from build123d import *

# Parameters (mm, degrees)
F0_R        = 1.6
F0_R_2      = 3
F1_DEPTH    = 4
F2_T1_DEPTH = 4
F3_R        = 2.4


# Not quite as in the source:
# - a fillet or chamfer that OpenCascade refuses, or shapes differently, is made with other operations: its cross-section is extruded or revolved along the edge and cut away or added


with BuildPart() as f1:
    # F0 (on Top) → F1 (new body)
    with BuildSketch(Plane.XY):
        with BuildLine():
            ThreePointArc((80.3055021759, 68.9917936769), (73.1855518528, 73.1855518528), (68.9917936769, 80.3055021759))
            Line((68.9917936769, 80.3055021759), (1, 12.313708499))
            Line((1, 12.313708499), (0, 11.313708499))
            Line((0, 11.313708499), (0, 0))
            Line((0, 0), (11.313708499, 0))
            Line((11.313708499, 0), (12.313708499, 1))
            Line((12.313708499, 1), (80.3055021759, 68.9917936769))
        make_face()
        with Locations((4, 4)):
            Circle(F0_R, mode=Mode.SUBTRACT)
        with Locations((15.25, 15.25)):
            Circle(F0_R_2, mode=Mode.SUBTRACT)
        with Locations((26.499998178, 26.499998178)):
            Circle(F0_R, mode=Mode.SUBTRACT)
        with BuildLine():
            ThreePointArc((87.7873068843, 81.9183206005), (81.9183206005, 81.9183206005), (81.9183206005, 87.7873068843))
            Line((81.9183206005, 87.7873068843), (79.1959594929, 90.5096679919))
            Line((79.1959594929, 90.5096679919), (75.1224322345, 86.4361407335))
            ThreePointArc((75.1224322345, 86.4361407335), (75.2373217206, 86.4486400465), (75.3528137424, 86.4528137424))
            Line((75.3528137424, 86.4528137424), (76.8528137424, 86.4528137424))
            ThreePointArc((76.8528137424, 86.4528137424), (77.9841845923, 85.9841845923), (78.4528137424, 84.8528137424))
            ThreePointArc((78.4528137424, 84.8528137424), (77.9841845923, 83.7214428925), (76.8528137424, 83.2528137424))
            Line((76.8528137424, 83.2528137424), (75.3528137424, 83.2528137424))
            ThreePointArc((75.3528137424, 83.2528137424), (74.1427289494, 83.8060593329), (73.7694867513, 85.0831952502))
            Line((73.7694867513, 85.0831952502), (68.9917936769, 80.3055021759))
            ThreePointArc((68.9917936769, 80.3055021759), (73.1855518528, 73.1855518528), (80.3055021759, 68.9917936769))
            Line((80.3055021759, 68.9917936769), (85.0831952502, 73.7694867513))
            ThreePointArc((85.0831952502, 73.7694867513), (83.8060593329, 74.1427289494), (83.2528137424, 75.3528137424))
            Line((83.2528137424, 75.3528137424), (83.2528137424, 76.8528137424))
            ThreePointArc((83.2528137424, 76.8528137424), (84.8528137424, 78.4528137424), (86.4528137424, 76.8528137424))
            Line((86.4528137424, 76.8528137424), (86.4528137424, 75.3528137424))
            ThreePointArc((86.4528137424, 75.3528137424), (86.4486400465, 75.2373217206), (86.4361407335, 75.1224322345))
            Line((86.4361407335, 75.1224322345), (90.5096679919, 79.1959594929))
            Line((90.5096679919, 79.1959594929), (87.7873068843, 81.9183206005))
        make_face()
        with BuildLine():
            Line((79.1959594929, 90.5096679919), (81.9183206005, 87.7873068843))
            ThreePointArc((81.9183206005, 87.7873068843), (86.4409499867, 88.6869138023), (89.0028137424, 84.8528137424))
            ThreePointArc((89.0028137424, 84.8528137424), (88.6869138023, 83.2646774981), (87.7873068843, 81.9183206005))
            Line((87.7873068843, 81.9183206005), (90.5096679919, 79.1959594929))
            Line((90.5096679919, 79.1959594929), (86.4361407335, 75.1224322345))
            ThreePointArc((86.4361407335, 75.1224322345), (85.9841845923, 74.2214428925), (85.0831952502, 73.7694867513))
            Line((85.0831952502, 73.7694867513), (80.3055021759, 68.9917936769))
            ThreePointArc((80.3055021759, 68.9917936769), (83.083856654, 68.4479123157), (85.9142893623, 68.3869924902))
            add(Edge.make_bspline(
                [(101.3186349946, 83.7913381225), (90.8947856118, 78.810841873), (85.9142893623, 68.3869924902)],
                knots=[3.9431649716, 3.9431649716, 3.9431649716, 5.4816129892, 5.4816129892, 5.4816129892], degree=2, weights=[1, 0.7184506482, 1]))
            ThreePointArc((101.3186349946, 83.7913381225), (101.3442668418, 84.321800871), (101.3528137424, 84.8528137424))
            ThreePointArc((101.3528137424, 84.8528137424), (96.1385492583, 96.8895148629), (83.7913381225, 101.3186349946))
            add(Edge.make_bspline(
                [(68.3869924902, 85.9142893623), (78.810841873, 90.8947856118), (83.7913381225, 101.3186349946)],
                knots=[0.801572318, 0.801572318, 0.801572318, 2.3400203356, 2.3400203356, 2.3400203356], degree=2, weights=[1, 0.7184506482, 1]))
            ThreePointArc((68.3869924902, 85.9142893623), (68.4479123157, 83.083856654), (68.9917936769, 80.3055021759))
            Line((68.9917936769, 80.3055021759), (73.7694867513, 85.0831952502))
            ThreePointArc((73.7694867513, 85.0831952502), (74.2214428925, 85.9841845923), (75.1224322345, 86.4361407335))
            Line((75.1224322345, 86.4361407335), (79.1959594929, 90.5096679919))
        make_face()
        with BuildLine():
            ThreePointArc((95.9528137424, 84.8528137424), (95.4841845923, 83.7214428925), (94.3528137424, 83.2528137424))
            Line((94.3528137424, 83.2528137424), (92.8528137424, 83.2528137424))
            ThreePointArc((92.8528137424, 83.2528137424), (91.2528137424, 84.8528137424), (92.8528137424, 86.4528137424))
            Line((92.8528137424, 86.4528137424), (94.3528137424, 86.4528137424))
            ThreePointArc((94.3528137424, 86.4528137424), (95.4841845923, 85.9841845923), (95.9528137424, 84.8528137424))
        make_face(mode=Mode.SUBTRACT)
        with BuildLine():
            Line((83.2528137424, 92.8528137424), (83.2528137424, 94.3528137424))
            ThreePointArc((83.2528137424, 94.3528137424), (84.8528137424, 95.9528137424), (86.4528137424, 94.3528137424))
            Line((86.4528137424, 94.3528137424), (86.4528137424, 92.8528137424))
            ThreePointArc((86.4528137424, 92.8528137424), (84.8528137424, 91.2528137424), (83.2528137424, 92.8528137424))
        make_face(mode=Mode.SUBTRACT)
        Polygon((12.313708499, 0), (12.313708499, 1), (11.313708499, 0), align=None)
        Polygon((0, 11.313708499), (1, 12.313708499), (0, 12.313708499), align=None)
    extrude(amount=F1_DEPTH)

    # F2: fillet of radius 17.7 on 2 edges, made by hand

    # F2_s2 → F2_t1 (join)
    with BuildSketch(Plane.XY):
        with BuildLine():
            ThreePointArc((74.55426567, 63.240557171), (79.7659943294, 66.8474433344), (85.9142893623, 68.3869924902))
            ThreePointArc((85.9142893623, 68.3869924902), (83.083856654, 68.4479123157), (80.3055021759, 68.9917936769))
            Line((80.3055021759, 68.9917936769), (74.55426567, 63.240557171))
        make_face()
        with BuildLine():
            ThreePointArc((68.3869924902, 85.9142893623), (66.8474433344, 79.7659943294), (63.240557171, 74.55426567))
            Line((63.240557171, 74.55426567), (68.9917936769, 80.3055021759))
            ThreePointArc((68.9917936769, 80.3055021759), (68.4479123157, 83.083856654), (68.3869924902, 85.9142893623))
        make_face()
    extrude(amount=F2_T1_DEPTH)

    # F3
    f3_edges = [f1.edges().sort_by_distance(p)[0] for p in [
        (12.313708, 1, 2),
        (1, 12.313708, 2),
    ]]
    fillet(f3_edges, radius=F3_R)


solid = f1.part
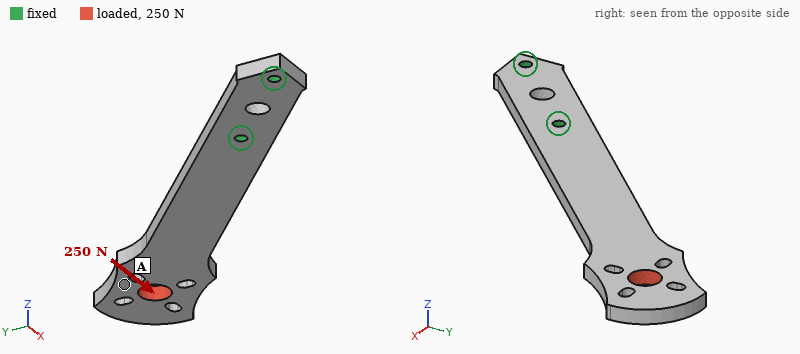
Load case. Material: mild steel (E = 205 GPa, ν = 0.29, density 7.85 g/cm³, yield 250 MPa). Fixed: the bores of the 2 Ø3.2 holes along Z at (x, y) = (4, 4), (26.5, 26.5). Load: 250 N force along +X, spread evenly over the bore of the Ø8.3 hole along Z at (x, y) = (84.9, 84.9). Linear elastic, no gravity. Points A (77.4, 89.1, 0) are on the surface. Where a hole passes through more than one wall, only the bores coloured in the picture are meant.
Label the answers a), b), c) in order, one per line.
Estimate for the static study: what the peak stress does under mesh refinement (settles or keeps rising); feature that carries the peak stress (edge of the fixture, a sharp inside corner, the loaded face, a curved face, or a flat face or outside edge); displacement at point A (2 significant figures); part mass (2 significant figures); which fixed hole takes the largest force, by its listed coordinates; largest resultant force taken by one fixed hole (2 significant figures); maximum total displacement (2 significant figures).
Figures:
a) keeps rising
b) edge of the fixture
c) 0.16 mm
d) 68 g
e) (26.5, 26.5)
f) 520 N
g) 0.20 mm
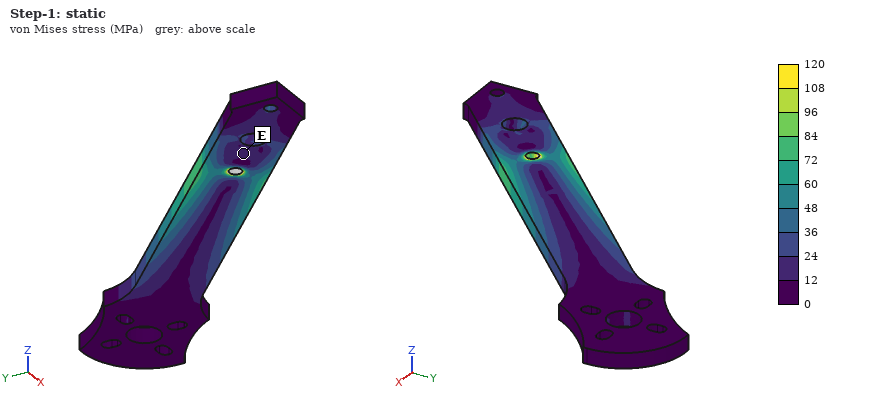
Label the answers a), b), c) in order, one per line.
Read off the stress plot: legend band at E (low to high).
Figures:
a) 12 to 24 MPa
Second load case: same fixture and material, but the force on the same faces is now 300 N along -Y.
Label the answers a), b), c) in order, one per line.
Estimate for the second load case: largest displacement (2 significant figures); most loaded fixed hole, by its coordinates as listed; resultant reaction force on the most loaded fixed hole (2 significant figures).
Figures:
a) 0.24 mm
b) (26.5, 26.5)
c) 620 N
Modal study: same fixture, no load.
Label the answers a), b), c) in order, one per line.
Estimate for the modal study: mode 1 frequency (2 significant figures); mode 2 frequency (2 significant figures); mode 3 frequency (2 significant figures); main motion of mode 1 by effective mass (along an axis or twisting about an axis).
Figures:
a) 320 Hz
b) 1100 Hz
c) 2100 Hz
d) along Z
